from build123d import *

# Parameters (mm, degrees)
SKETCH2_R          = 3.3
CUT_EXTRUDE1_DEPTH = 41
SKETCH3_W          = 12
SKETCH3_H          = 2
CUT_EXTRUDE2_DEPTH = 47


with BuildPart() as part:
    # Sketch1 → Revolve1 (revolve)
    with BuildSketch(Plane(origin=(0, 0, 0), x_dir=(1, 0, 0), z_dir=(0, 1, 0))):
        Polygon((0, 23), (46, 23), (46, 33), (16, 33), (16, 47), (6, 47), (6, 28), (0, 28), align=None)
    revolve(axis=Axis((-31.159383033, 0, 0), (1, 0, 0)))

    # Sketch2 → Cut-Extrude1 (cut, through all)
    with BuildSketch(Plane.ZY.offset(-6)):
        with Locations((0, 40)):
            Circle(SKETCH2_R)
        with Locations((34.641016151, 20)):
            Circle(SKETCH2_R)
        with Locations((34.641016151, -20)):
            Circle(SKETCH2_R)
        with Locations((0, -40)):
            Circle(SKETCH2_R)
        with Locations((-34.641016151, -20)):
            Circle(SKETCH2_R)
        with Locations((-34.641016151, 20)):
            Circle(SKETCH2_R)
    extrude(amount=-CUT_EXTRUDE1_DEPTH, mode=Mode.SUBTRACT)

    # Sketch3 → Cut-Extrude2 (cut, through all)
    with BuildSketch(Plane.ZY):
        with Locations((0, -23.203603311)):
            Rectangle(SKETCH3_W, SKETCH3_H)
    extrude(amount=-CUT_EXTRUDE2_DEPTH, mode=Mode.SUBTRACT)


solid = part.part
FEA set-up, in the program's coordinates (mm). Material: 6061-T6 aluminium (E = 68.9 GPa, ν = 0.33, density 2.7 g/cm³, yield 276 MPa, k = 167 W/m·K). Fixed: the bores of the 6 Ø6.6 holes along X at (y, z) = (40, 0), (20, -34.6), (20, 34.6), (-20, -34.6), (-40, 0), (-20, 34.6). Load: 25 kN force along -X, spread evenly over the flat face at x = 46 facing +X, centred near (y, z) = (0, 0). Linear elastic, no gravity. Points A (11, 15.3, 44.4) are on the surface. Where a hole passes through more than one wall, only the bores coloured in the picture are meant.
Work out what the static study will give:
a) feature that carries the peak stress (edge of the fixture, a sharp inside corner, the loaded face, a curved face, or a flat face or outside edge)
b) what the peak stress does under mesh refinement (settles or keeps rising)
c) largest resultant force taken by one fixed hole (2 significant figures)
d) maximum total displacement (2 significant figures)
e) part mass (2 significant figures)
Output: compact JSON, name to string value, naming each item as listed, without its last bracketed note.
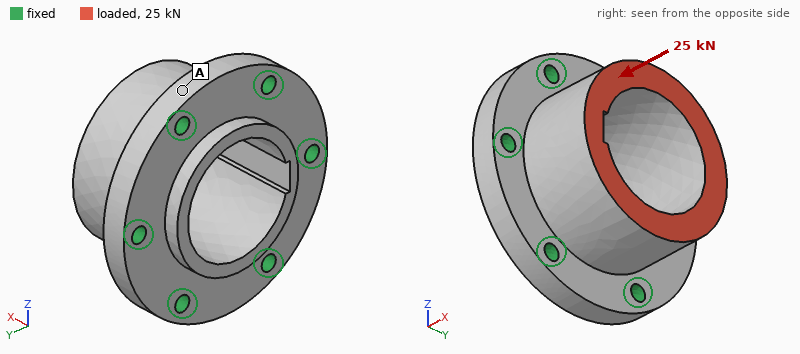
{"feature that carries the peak stress": "edge of the fixture", "what the peak stress does under mesh refinement": "keeps rising", "largest resultant force taken by one fixed hole": "4.4 kN", "maximum total displacement": "18 µm", "part mass": "290 g"}
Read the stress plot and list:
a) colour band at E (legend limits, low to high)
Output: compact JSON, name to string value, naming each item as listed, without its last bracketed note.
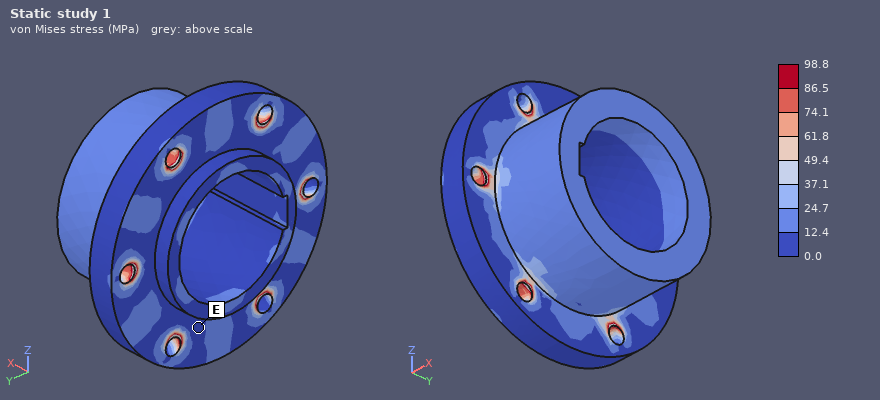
{"colour band at E": "0.0 to 12.4 MPa"}
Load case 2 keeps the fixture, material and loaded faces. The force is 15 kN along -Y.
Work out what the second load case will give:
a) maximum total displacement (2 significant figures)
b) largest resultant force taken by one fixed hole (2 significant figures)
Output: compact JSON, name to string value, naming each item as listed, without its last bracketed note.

{"maximum total displacement": "51 µm", "largest resultant force taken by one fixed hole": "5.6 kN"}
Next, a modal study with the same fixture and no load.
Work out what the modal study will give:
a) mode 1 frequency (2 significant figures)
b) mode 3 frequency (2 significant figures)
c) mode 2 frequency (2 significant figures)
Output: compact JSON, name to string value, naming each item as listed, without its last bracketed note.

{"mode 1 frequency": "12 kHz", "mode 3 frequency": "13 kHz", "mode 2 frequency": "13 kHz"}
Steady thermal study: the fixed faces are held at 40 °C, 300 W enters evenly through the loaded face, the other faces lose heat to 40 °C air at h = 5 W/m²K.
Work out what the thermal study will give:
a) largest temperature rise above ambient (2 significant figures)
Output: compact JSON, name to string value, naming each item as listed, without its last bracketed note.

{"largest temperature rise above ambient": "45 K"}
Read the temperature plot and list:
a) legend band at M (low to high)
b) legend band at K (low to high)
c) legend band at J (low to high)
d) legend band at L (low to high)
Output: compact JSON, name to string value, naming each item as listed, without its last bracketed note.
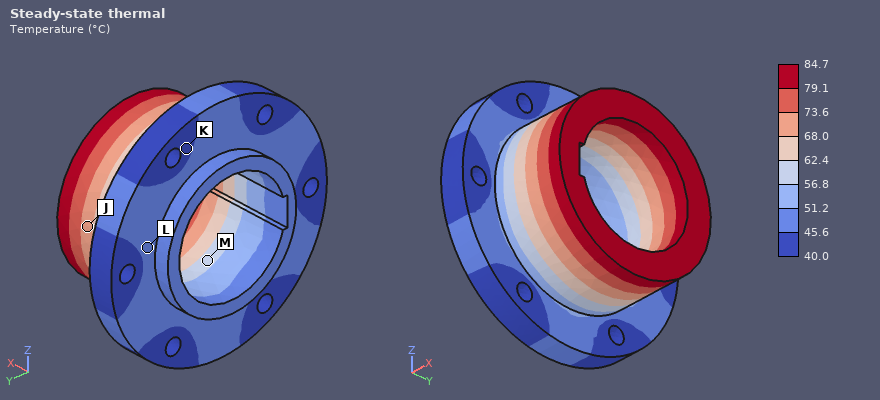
{"legend band at M": "56.8 to 62.4 °C", "legend band at K": "40.0 to 45.6 °C", "legend band at J": "68.0 to 73.6 °C", "legend band at L": "45.6 to 51.2 °C"}
